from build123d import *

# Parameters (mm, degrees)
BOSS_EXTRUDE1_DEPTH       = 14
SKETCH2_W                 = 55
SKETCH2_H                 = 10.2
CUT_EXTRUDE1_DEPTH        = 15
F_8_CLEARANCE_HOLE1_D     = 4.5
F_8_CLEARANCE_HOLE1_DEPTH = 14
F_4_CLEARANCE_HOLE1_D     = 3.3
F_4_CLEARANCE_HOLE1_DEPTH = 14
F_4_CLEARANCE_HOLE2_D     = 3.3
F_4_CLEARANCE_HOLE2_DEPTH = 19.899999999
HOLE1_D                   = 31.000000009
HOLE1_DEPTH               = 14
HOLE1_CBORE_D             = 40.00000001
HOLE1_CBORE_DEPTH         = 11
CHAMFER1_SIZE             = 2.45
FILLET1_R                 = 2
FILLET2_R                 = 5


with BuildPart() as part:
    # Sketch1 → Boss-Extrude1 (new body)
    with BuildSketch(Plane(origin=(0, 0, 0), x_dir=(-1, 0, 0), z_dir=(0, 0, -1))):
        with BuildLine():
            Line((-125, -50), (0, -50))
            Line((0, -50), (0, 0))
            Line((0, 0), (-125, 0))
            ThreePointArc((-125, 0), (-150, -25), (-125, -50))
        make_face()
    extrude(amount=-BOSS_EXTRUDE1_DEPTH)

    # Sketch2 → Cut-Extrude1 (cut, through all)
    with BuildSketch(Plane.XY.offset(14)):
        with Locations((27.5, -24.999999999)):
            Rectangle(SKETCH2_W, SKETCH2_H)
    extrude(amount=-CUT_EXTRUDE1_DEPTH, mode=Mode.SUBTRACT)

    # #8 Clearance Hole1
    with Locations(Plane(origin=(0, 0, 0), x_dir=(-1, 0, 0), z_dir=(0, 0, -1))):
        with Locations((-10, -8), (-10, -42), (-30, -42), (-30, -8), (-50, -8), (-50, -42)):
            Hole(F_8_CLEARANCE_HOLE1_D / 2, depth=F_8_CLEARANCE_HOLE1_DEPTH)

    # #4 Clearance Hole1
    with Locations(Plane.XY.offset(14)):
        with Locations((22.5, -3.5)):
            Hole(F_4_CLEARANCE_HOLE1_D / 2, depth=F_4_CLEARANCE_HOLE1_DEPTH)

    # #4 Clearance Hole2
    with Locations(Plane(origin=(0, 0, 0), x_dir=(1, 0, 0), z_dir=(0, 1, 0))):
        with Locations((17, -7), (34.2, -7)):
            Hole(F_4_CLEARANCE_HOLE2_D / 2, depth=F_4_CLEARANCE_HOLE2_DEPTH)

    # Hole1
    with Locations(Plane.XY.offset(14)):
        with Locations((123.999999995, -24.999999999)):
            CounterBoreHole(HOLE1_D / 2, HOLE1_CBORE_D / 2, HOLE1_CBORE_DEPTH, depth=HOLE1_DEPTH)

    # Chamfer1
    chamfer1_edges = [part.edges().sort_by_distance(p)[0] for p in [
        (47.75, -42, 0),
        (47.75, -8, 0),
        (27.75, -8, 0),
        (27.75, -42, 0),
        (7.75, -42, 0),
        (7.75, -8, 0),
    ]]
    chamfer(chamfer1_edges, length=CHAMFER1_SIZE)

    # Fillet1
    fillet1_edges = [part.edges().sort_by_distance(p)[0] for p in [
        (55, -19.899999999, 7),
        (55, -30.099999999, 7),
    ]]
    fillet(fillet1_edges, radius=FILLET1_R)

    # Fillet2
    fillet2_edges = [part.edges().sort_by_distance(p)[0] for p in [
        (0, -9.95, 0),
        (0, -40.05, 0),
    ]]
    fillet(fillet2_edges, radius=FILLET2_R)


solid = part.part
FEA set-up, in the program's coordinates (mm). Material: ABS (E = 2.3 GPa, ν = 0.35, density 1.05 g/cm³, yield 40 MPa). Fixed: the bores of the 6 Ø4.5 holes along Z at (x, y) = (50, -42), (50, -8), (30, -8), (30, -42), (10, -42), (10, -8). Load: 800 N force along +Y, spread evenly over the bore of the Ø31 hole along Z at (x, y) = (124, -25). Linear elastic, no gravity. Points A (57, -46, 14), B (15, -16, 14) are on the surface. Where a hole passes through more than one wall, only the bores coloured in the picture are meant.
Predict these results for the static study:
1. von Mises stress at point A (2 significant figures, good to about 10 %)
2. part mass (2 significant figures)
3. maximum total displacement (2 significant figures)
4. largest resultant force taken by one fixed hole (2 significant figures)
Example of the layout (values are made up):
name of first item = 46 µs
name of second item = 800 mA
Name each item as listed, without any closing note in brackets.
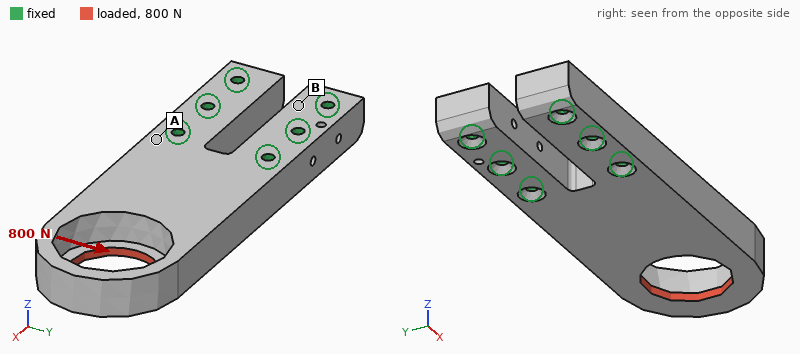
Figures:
von Mises stress at point A = 9.1 MPa
part mass = 79 g
maximum total displacement = 1.2 mm
largest resultant force taken by one fixed hole = 1.5 kN
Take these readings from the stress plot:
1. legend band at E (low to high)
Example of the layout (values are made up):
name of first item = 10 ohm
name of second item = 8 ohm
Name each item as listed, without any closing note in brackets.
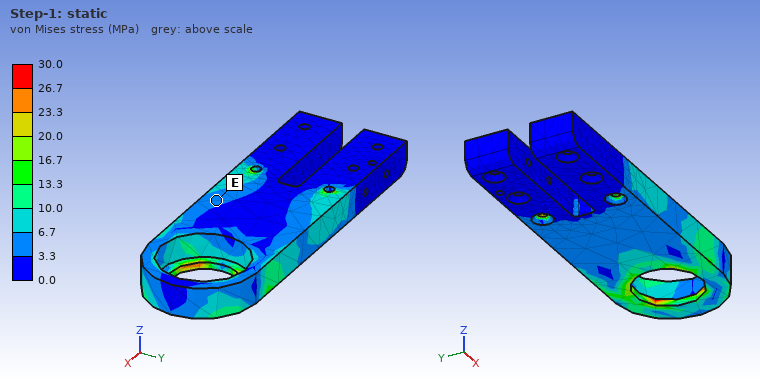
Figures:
legend band at E = 3.3 to 6.7 MPa
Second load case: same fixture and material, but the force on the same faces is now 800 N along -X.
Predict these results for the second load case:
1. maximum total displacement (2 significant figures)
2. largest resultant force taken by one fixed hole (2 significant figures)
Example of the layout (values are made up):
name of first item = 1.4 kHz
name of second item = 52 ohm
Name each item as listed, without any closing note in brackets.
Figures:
maximum total displacement = 1.1 mm
largest resultant force taken by one fixed hole = 320 N
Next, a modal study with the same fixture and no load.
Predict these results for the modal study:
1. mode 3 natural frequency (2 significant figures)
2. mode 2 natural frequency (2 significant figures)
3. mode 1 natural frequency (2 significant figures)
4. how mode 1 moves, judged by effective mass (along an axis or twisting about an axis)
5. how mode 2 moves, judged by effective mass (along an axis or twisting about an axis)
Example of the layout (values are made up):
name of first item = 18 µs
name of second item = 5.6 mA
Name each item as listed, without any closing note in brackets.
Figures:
mode 3 natural frequency = 1400 Hz
mode 2 natural frequency = 1200 Hz
mode 1 natural frequency = 440 Hz
how mode 1 moves, judged by effective mass = along Z
how mode 2 moves, judged by effective mass = along Y
